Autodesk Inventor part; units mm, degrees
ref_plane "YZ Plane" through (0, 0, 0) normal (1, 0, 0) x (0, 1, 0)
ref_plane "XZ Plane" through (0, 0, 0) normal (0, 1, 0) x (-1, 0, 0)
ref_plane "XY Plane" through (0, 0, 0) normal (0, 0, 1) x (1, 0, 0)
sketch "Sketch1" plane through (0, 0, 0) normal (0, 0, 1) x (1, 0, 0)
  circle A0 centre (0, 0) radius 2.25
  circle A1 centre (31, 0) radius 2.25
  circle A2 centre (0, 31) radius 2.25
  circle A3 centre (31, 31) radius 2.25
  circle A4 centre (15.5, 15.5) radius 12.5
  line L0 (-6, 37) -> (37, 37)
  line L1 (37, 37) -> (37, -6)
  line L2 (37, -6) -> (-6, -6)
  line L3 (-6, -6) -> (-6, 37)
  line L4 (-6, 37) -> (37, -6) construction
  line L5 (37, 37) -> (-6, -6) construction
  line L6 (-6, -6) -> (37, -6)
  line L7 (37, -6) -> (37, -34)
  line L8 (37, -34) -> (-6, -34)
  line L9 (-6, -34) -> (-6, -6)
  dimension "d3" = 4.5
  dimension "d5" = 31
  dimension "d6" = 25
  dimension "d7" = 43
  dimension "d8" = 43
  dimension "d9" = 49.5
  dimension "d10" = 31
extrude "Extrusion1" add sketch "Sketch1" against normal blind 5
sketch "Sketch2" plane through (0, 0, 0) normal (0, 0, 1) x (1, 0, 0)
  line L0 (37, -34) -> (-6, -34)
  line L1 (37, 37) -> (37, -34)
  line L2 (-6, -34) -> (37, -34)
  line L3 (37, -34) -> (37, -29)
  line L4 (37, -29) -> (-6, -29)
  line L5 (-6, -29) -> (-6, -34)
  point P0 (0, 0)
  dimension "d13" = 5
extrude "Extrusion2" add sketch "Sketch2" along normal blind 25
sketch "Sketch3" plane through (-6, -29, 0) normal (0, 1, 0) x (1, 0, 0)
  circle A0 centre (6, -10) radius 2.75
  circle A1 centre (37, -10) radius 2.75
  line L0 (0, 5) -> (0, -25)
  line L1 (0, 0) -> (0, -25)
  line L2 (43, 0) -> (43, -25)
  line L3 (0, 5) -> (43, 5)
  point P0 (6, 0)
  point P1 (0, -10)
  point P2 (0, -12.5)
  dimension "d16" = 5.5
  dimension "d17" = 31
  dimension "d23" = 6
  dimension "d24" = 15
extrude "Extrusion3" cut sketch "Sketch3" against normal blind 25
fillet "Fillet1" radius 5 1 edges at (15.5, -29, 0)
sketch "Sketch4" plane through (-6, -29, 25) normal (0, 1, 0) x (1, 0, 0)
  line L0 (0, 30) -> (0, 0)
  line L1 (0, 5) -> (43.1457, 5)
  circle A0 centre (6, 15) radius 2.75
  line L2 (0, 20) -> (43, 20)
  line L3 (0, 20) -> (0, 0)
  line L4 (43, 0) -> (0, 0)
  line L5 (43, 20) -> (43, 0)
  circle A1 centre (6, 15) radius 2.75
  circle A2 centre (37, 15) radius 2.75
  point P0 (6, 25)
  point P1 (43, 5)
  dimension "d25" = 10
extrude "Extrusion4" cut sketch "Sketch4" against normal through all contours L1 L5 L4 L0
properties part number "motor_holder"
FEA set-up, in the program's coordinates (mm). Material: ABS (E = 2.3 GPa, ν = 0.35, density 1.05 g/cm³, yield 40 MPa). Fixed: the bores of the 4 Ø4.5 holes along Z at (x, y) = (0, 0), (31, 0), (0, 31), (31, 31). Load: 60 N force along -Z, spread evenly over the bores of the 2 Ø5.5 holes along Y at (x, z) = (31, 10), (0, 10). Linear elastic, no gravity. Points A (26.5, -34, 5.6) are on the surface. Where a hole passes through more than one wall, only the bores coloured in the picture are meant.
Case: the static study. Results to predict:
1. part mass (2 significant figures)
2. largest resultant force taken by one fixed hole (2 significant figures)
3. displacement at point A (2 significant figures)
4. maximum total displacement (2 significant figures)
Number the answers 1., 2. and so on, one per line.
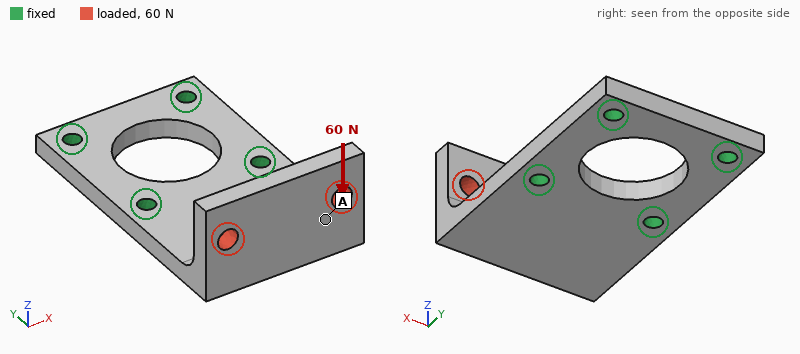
1. 18 g
2. 33 N
3. 0.76 mm
4. 0.97 mm
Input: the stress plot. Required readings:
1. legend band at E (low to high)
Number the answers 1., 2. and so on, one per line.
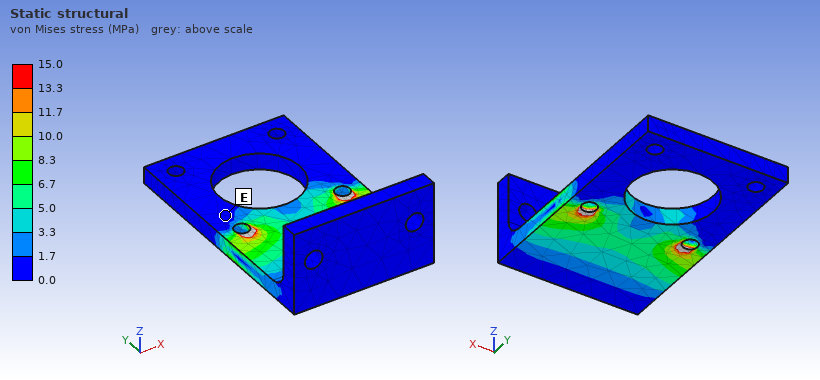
1. 0.0 to 1.7 MPa
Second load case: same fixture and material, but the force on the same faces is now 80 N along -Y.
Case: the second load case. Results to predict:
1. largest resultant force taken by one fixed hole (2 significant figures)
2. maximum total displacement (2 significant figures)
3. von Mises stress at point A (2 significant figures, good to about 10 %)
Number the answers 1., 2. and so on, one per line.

1. 40 N
2. 0.88 mm
3. 1.7 MPa
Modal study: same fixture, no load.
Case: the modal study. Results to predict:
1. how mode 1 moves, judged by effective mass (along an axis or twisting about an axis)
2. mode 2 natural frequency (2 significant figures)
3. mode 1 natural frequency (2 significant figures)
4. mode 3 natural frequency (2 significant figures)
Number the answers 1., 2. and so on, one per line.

1. along Z
2. 1100 Hz
3. 520 Hz
4. 2000 Hz
